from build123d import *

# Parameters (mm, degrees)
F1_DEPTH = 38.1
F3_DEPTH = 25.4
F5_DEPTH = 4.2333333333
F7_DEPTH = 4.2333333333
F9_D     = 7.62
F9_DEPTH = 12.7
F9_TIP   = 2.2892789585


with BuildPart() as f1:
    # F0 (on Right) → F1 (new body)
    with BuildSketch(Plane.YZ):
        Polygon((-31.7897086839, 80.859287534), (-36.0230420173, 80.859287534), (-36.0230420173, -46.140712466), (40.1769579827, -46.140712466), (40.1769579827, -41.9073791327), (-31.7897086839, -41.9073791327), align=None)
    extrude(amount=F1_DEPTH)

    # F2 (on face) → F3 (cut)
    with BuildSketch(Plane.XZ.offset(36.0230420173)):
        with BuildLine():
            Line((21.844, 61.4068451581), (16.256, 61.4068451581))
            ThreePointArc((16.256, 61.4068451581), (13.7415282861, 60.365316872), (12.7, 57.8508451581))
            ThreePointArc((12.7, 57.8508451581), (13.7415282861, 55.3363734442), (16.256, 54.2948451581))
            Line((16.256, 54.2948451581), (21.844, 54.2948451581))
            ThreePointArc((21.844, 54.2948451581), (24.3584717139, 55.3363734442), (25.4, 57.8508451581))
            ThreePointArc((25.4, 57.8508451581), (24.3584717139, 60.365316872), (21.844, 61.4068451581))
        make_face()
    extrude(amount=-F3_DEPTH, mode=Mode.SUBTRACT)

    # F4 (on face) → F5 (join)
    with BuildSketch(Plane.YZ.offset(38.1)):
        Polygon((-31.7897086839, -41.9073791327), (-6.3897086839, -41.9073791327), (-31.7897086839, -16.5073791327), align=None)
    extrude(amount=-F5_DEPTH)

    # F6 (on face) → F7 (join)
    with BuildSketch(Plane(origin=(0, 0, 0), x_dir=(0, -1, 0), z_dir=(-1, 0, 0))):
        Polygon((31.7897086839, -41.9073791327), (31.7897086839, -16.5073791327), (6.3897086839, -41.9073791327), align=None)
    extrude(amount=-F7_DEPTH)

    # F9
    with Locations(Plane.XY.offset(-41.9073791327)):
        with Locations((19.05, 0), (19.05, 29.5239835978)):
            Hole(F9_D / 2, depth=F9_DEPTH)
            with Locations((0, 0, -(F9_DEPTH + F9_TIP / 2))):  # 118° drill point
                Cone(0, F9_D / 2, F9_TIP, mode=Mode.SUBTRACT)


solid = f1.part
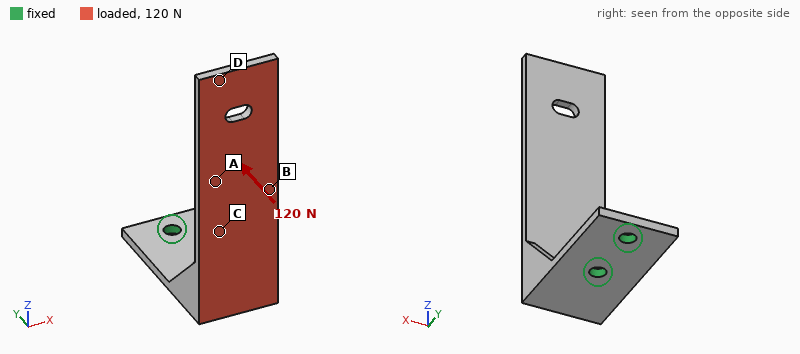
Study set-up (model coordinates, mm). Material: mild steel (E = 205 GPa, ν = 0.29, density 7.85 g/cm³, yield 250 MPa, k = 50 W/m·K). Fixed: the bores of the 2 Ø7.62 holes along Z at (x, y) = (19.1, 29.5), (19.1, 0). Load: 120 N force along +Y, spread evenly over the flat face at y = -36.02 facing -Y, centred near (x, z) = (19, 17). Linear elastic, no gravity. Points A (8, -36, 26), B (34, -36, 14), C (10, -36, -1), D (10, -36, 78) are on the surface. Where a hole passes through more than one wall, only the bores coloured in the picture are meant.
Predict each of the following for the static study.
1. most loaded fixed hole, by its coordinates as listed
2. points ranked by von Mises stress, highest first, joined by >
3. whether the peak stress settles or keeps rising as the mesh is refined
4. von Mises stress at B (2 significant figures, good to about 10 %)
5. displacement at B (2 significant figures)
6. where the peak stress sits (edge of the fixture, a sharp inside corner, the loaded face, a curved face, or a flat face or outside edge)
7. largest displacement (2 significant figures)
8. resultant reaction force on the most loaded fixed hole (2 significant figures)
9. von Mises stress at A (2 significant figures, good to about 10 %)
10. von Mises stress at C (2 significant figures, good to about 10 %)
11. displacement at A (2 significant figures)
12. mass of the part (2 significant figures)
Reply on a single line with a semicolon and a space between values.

(19.1, 29.5); C > B > A > D; keeps rising; 19 MPa; 0.17 mm; edge of the fixture; 0.52 mm; 90 N; 13 MPa; 28 MPa; 0.23 mm; 270 g
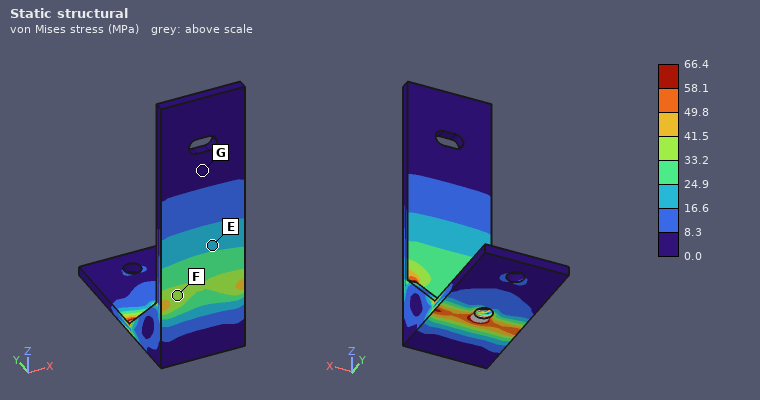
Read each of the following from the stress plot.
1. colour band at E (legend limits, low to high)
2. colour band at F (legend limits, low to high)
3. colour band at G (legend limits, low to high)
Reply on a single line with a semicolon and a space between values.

16.6 to 24.9 MPa; 33.2 to 41.5 MPa; 0.0 to 8.3 MPa
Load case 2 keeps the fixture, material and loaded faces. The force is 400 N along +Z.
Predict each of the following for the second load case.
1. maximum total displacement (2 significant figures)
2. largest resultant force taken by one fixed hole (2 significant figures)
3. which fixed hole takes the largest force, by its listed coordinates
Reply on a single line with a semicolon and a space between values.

0.41 mm; 510 N; (19.1, 0)
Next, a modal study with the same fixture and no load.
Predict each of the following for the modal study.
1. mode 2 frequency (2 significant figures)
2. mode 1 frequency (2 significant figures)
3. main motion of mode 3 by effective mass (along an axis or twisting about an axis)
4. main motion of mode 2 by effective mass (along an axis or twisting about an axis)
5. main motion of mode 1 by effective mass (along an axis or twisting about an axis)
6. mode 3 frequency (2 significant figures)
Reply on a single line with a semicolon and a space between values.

380 Hz; 240 Hz; along Z; along X; along Y; 930 Hz
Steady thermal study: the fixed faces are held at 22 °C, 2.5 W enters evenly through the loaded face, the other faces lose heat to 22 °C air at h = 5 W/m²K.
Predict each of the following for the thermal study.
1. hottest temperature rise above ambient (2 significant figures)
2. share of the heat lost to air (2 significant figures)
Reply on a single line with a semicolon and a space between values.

19 K; 22 %
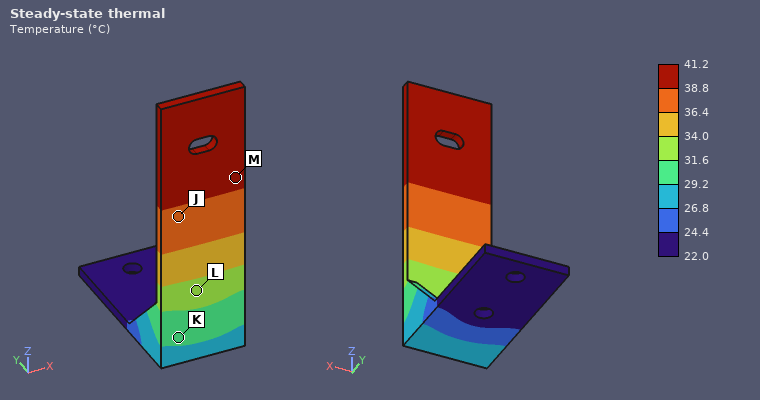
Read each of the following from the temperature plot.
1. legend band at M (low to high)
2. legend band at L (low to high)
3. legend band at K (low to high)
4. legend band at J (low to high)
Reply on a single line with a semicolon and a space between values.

38.8 to 41.2 °C; 31.6 to 34.0 °C; 29.2 to 31.6 °C; 36.4 to 38.8 °C
